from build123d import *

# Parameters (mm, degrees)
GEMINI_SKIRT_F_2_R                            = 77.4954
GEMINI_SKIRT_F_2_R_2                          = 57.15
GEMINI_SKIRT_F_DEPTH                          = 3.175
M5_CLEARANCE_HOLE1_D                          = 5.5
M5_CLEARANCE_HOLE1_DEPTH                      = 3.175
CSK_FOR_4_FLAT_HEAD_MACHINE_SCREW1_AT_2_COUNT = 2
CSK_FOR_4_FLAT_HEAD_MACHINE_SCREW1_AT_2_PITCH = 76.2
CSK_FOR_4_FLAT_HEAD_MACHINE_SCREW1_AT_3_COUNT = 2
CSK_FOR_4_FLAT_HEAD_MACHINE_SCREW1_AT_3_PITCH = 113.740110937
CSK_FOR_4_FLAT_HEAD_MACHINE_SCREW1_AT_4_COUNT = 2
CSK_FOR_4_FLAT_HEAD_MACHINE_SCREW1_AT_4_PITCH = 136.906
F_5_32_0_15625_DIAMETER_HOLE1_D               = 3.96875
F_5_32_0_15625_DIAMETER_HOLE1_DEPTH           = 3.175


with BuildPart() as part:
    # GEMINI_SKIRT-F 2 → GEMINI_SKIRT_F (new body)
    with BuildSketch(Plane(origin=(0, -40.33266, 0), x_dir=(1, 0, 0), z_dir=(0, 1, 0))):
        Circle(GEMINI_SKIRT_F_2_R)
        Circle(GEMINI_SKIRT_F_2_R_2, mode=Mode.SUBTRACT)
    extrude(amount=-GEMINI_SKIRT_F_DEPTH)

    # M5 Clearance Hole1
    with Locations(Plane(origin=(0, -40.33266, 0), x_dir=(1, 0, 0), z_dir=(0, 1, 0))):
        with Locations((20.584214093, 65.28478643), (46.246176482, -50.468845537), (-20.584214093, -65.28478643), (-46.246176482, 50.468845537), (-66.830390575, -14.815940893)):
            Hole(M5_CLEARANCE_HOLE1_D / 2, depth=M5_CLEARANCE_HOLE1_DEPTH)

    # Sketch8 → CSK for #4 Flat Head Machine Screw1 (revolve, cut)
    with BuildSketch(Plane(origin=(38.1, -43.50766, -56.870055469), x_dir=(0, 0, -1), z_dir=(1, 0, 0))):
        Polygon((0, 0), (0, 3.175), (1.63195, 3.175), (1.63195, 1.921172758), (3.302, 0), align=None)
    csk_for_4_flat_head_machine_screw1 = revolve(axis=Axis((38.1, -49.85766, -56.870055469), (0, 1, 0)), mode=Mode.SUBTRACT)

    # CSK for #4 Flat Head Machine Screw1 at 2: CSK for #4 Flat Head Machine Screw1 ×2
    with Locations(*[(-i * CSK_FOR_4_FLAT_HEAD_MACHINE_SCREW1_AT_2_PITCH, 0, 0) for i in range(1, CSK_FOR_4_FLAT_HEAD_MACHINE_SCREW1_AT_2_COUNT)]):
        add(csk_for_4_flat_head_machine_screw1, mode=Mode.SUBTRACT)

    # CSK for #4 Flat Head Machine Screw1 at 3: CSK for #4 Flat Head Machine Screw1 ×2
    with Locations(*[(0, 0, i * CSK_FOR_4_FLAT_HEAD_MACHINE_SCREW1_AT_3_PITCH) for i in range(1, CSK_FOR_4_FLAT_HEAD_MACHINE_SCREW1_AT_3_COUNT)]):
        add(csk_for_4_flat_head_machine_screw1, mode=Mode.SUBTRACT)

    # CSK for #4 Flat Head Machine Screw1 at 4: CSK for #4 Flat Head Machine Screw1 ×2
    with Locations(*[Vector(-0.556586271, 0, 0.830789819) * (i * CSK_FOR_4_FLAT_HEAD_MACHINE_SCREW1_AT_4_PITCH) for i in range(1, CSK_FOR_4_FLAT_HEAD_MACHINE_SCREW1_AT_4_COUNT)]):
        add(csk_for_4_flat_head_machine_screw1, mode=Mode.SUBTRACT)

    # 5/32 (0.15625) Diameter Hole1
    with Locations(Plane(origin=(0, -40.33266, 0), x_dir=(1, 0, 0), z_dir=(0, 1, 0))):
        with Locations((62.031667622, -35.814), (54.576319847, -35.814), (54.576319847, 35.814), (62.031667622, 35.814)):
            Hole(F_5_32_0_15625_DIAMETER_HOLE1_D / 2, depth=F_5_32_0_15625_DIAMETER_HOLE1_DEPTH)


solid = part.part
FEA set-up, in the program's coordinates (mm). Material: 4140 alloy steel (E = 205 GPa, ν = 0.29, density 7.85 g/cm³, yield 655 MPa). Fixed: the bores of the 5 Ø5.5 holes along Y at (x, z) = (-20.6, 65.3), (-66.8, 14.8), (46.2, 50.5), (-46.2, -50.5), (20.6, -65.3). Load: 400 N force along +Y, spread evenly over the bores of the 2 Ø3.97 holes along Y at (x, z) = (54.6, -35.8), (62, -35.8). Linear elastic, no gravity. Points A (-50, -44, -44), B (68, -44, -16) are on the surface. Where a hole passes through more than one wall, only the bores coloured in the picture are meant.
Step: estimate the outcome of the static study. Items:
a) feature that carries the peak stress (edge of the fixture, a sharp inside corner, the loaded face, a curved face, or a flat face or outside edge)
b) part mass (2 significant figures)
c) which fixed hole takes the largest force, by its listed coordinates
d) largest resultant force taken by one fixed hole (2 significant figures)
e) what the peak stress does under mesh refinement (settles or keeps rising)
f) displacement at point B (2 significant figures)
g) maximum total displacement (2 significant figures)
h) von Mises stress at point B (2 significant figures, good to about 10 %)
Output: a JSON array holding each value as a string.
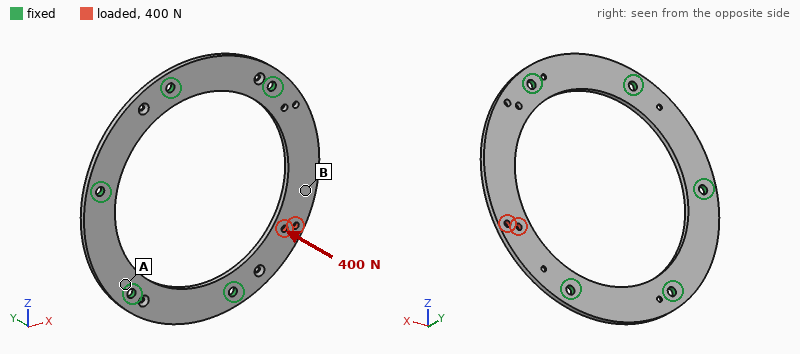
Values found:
["edge of the fixture", "210 g", "(20.6, -65.3)", "310 N", "keeps rising", "0.55 mm", "0.65 mm", "82 MPa"]
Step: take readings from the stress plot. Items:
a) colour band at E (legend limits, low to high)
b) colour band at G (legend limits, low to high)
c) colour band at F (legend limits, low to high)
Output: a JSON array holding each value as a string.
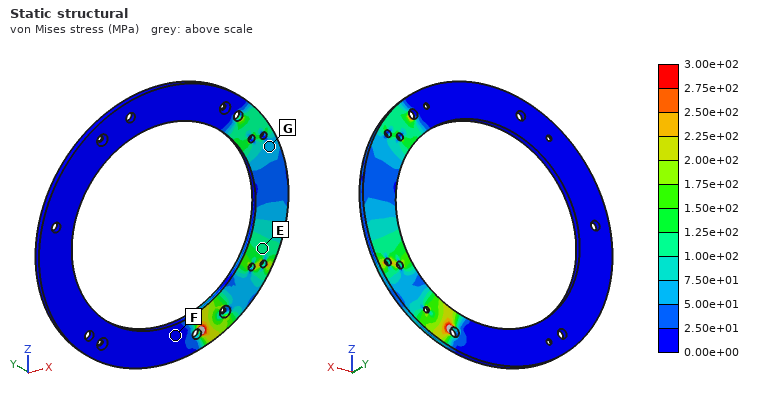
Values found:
["1.00e+02 to 1.25e+02 MPa", "5.00e+01 to 7.50e+01 MPa", "0.00e+00 to 2.50e+01 MPa"]
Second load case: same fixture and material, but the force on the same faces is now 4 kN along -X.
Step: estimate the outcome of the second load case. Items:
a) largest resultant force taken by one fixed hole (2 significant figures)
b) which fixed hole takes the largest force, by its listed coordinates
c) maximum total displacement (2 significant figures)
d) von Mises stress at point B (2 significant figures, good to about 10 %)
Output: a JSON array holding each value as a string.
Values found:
["3.9 kN", "(20.6, -65.3)", "42 µm", "42 MPa"]
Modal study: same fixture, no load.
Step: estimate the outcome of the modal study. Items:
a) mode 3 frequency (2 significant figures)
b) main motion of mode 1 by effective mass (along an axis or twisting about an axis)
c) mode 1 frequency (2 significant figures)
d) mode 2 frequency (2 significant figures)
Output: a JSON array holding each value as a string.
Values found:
["3300 Hz", "along Y", "750 Hz", "2200 Hz"]
